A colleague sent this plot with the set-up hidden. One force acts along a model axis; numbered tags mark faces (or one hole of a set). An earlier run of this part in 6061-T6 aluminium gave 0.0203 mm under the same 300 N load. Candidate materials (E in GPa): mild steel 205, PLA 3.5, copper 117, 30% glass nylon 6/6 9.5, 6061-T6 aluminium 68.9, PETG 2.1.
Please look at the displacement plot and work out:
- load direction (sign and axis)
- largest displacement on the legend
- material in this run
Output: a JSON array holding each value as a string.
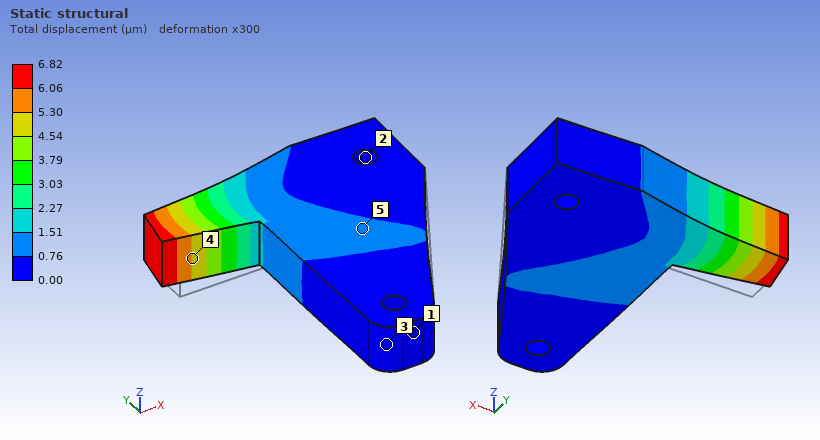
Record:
["+Y", "6.82 µm", "mild steel"]
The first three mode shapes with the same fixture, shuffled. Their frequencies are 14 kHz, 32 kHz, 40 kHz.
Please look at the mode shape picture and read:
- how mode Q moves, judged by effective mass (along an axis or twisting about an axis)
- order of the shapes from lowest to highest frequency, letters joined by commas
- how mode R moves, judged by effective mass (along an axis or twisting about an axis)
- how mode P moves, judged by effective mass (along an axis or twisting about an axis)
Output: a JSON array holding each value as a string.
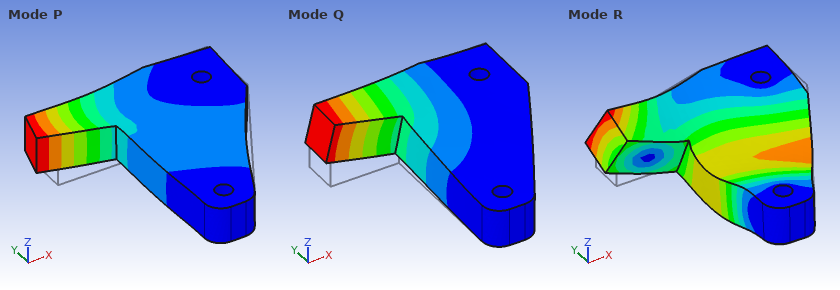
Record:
["along Z", "Q, P, R", "along Z", "along Y"]
